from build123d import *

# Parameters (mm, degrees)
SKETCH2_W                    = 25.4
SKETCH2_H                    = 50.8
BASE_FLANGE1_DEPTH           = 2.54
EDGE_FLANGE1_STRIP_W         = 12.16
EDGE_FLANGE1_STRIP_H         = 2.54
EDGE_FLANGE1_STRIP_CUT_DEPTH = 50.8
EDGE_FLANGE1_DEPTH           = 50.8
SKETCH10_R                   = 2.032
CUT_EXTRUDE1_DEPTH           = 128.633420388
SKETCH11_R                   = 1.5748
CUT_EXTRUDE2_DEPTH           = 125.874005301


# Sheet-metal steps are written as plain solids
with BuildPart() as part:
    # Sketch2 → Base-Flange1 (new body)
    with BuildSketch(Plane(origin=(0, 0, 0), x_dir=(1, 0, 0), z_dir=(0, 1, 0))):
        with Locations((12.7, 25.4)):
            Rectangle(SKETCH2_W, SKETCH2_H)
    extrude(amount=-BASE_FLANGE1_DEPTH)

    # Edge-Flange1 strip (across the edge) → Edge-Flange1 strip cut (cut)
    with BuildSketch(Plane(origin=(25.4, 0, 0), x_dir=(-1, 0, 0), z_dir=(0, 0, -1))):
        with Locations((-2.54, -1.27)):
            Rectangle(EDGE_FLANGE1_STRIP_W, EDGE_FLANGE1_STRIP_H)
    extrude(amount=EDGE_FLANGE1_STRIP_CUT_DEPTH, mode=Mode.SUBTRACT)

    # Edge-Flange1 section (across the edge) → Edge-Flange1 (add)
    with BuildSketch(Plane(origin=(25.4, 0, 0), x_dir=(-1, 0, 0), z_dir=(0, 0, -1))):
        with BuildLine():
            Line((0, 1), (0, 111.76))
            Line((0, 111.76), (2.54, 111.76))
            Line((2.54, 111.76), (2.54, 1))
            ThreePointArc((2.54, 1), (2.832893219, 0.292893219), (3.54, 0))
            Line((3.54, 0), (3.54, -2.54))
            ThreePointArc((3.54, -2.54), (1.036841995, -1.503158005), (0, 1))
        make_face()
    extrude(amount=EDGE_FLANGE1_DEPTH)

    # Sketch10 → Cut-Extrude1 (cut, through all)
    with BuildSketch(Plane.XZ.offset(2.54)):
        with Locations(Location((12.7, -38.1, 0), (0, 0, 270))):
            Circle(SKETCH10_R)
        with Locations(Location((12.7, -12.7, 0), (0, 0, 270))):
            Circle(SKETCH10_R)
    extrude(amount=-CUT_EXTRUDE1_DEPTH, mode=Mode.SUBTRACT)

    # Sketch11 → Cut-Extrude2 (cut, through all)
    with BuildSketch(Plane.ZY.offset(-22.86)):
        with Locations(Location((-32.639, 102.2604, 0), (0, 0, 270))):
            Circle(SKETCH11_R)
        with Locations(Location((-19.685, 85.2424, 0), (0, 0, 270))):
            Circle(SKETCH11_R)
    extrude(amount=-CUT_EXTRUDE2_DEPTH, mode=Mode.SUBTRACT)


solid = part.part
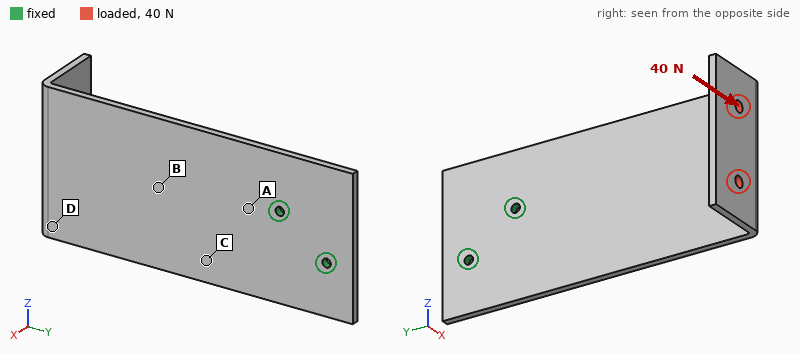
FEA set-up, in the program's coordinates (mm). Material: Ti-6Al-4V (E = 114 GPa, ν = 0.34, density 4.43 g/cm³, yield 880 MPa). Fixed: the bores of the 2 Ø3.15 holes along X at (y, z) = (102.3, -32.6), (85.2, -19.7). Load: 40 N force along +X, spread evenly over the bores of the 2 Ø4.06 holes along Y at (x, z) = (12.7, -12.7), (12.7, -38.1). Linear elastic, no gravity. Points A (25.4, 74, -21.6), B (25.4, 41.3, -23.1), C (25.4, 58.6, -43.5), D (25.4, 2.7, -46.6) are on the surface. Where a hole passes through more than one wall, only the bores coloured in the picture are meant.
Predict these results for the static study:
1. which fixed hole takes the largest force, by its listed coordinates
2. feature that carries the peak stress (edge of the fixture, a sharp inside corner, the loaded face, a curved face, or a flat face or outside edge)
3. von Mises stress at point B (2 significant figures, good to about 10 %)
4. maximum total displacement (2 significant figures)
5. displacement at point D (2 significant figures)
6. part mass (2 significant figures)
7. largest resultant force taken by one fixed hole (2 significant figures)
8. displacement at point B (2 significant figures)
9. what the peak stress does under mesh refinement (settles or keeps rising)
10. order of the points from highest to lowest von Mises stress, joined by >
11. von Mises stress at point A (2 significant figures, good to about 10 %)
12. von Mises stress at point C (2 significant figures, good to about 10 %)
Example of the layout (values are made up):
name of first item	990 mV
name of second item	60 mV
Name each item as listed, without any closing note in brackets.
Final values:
which fixed hole takes the largest force, by its listed coordinates	(85.2, -19.7)
feature that carries the peak stress	edge of the fixture
von Mises stress at point B	29 MPa
maximum total displacement	1.3 mm
displacement at point D	1.1 mm
part mass	77 g
largest resultant force taken by one fixed hole	110 N
displacement at point B	0.40 mm
what the peak stress does under mesh refinement	keeps rising
order of the points from highest to lowest von Mises stress, joined by >	A > C > B > D
von Mises stress at point A	54 MPa
von Mises stress at point C	42 MPa
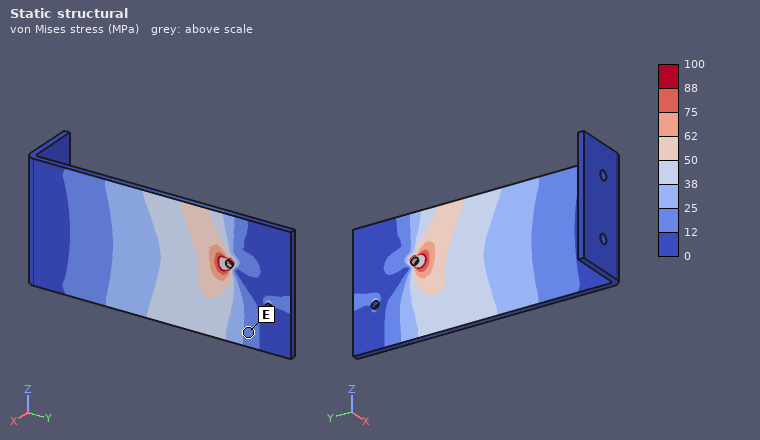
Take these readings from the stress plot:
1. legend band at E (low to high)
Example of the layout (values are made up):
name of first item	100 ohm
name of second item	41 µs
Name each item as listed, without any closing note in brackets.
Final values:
legend band at E	12 to 25 MPa
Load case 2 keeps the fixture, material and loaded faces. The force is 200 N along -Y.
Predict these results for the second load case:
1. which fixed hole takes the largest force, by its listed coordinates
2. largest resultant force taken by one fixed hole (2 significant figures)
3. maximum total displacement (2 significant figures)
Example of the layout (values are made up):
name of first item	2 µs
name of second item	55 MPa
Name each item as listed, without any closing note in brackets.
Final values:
which fixed hole takes the largest force, by its listed coordinates	(85.2, -19.7)
largest resultant force taken by one fixed hole	130 N
maximum total displacement	1.3 mm
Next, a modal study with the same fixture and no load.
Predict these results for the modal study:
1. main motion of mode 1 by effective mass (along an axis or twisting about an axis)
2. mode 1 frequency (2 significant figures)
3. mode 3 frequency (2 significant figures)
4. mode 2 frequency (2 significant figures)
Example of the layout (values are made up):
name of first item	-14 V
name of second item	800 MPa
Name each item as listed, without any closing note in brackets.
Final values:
main motion of mode 1 by effective mass	along X
mode 1 frequency	180 Hz
mode 3 frequency	1100 Hz
mode 2 frequency	600 Hz
